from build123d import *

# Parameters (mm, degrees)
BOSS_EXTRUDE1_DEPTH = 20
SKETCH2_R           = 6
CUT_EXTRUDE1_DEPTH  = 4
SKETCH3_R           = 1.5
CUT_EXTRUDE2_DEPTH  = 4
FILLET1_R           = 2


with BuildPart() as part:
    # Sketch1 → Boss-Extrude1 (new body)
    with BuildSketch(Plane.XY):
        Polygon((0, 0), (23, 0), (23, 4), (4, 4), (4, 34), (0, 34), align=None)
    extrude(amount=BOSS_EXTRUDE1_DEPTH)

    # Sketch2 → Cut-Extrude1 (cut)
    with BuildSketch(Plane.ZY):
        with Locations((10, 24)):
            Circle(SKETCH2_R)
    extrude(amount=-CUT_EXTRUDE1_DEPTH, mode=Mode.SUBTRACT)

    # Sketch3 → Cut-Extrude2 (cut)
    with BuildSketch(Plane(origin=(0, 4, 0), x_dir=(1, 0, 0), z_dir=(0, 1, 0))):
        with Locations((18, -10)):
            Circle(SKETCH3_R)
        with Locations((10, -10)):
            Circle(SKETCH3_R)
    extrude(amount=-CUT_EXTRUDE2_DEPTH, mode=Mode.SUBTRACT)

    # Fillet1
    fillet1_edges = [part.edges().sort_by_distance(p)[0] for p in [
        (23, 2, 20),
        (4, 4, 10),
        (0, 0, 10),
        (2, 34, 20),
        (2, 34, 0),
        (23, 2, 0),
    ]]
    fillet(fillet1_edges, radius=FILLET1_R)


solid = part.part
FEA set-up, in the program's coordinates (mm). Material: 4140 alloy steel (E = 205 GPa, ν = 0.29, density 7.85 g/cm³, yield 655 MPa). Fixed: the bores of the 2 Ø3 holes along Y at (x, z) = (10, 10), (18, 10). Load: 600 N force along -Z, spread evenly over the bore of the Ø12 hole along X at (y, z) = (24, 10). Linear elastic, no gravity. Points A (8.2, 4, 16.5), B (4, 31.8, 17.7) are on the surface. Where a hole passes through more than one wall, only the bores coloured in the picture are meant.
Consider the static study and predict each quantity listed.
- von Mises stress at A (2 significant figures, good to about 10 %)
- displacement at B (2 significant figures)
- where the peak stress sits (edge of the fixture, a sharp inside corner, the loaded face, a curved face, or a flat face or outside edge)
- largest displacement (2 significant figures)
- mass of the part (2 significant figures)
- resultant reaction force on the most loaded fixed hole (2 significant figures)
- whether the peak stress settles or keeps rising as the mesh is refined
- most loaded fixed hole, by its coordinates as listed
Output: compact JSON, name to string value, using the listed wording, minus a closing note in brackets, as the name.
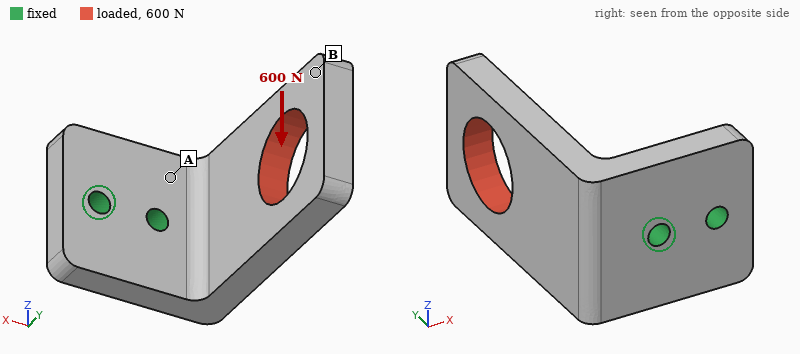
{"von Mises stress at A": "100 MPa", "displacement at B": "0.10 mm", "where the peak stress sits": "edge of the fixture", "largest displacement": "0.11 mm", "mass of the part": "29 g", "resultant reaction force on the most loaded fixed hole": "970 N", "whether the peak stress settles or keeps rising as the mesh is refined": "keeps rising", "most loaded fixed hole, by its coordinates as listed": "(10, 10)"}
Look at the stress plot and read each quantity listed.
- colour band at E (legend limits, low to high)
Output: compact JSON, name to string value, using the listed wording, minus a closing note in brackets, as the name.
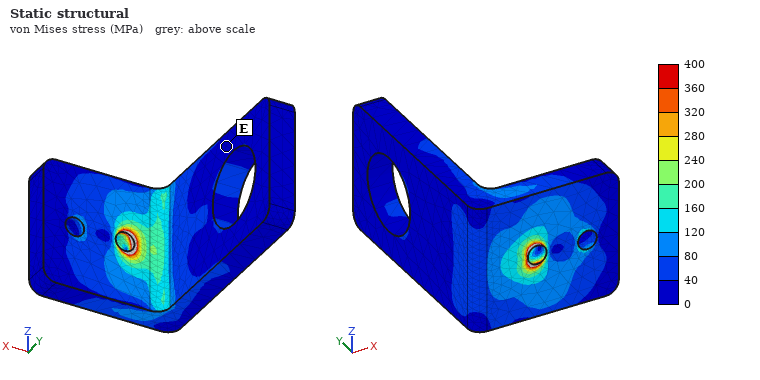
{"colour band at E": "0 to 40 MPa"}
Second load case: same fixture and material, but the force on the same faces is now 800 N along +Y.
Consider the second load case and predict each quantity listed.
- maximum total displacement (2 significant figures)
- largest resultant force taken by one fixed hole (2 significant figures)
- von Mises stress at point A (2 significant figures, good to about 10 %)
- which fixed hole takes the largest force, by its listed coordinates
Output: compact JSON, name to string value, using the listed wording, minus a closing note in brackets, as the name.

{"maximum total displacement": "46 µm", "largest resultant force taken by one fixed hole": "1.0 kN", "von Mises stress at point A": "55 MPa", "which fixed hole takes the largest force, by its listed coordinates": "(10, 10)"}
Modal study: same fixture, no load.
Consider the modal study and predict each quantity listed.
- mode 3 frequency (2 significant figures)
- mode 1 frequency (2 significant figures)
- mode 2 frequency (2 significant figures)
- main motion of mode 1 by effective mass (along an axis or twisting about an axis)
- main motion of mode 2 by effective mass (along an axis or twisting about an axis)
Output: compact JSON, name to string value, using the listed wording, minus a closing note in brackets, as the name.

{"mode 3 frequency": "9200 Hz", "mode 1 frequency": "2800 Hz", "mode 2 frequency": "4300 Hz", "main motion of mode 1 by effective mass": "along X", "main motion of mode 2 by effective mass": "along Z"}
